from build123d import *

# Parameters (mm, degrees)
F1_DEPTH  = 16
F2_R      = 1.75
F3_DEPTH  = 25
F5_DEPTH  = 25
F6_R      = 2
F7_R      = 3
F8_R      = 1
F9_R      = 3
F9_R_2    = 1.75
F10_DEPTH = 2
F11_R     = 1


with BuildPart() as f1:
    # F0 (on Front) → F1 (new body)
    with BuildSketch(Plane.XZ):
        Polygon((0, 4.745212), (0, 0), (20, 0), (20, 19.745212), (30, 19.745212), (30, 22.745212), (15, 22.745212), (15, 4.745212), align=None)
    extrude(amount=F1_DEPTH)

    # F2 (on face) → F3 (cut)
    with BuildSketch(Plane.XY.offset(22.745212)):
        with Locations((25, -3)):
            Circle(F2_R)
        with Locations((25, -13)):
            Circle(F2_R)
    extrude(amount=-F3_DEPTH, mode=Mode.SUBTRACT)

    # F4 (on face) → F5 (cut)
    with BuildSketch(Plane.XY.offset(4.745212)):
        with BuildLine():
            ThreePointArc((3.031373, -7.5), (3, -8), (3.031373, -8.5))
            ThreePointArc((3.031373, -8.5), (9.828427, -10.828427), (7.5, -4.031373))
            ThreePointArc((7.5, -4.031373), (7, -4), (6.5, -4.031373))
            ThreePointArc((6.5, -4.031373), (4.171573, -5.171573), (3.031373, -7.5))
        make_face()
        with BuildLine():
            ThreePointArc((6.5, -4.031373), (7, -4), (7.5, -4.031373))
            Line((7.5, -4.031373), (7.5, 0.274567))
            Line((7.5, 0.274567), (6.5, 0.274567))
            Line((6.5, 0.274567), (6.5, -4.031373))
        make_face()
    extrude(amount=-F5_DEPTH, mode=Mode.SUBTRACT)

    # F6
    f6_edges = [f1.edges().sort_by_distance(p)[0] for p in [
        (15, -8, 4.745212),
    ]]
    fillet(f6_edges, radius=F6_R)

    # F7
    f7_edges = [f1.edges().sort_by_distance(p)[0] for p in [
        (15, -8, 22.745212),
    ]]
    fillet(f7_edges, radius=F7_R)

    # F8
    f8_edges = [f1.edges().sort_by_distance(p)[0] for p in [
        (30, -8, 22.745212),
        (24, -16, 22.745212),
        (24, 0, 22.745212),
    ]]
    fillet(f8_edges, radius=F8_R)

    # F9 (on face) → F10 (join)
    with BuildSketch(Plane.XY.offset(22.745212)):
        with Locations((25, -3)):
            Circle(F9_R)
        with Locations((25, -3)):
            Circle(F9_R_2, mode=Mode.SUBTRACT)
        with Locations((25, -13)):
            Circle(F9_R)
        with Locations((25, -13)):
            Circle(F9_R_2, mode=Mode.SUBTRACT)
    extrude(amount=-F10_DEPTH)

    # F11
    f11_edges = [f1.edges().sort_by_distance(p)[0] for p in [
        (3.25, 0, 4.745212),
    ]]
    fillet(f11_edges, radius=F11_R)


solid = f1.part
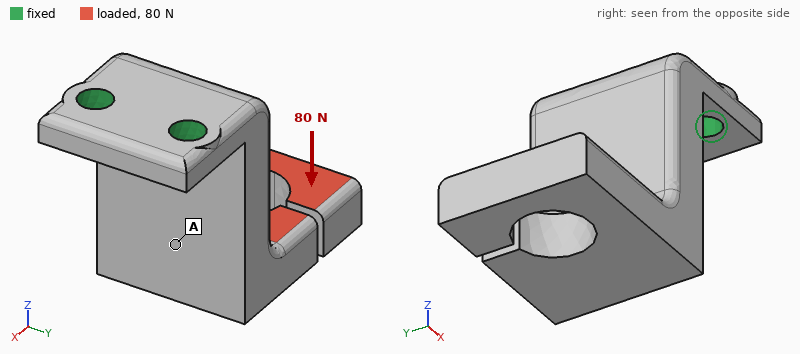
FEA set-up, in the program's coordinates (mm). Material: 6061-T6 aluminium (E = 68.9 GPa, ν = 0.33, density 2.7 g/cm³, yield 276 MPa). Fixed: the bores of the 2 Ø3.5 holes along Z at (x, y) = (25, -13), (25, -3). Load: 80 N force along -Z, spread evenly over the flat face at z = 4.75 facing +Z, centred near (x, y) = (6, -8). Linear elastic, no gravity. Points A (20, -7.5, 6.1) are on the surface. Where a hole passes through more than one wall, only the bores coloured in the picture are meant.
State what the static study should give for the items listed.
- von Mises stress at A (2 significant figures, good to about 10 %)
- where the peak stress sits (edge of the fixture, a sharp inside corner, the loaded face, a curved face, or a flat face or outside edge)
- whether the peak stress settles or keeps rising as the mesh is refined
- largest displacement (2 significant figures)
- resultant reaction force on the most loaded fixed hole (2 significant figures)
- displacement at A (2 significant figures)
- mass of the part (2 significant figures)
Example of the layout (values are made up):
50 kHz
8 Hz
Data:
10 MPa
edge of the fixture
keeps rising
0.14 mm
42 N
0.047 mm
8.3 g
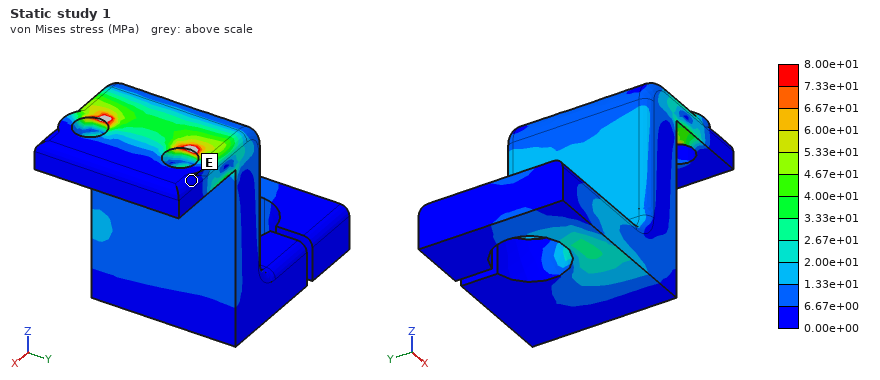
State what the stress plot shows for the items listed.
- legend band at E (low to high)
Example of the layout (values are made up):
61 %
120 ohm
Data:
0.00e+00 to 6.67e+00 MPa
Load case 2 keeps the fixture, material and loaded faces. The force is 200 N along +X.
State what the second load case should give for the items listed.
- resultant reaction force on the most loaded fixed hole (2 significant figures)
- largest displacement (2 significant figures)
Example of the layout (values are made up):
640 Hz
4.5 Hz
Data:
110 N
0.29 mm
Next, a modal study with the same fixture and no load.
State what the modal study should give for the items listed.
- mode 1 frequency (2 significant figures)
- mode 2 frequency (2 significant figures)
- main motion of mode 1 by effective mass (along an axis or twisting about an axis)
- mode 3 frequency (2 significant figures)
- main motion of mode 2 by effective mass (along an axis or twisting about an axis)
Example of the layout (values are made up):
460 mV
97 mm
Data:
2100 Hz
5100 Hz
along X
6700 Hz
along Y
